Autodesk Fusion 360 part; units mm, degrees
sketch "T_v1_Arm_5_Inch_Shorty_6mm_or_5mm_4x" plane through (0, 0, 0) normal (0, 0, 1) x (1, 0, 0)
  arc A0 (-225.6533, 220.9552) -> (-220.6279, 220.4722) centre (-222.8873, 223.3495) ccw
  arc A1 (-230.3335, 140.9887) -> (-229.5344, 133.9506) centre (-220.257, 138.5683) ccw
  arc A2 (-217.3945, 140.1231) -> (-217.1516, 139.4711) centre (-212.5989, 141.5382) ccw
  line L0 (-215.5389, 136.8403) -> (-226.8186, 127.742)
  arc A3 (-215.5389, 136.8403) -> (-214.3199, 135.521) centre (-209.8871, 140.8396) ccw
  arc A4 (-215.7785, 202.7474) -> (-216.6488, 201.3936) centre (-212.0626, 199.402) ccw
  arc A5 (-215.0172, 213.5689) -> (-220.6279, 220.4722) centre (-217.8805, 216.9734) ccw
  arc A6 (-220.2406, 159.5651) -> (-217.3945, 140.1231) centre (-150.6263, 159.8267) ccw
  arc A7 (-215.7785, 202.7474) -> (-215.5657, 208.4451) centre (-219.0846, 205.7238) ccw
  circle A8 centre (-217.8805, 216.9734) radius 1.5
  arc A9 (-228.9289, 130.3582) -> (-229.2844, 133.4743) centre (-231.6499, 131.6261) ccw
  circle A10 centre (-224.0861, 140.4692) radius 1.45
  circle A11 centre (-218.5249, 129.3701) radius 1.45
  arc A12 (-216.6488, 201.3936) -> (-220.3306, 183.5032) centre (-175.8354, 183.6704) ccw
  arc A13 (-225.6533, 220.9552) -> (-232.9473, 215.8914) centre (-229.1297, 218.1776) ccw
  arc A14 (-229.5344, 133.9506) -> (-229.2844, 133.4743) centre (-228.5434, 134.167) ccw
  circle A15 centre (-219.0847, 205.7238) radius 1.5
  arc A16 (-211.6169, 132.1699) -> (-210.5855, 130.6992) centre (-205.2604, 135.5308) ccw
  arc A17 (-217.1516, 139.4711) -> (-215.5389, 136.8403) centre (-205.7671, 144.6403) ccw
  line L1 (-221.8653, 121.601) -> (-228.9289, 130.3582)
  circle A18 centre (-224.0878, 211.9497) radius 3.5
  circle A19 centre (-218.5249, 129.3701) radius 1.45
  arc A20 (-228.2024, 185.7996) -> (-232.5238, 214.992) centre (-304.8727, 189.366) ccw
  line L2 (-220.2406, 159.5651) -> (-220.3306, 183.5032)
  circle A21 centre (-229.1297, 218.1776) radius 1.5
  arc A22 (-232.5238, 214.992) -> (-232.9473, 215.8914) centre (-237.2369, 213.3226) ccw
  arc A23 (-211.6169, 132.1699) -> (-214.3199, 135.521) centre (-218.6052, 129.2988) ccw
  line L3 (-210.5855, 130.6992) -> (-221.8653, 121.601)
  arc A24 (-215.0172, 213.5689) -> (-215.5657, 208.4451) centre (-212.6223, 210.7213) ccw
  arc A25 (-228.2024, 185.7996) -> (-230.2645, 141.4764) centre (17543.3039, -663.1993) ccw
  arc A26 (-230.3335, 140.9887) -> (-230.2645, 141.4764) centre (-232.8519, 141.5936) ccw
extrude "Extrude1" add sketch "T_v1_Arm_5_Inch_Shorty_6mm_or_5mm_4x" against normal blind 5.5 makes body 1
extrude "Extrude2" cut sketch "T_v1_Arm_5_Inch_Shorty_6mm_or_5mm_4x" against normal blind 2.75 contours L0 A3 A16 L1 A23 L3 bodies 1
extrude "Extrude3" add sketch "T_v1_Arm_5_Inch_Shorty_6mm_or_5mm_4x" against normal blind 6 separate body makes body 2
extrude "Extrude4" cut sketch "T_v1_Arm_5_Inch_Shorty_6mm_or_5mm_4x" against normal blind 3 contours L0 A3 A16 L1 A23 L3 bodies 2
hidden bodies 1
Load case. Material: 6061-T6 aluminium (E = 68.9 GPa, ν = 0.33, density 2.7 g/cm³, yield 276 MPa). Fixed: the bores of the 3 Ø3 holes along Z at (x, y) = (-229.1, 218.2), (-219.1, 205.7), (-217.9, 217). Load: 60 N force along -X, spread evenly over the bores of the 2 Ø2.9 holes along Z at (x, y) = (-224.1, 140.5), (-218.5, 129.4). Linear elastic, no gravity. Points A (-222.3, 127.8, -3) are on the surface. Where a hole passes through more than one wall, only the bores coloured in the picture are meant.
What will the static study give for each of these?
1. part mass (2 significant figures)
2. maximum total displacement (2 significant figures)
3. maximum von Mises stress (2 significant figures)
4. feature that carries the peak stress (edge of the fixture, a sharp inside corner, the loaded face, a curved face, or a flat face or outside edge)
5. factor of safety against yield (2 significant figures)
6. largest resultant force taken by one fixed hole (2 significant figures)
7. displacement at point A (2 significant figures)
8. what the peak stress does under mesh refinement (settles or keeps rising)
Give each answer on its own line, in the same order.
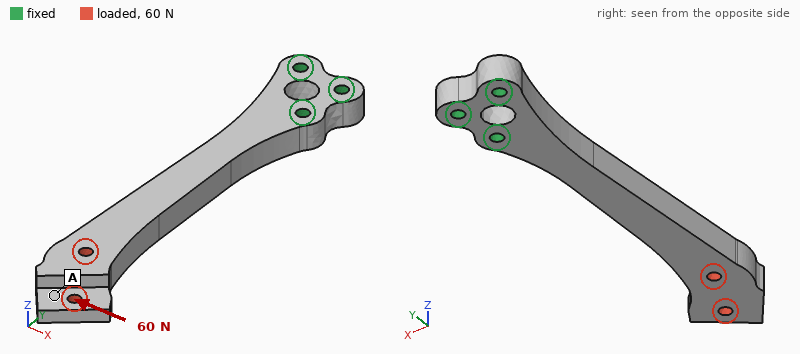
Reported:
16 g
0.35 mm
49 MPa
a curved face
5.7
300 N
0.31 mm
settles
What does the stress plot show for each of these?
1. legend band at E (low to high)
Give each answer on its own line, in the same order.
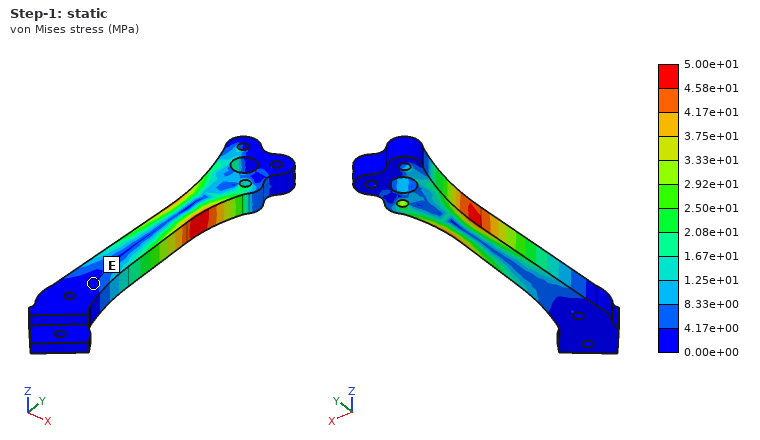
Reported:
0.00e+00 to 4.17e+00 MPa
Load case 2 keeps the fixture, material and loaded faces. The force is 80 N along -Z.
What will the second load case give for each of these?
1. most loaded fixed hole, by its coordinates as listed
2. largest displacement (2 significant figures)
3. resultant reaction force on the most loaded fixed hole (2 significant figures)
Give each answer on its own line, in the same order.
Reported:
(-219.1, 205.7)
1.0 mm
230 N
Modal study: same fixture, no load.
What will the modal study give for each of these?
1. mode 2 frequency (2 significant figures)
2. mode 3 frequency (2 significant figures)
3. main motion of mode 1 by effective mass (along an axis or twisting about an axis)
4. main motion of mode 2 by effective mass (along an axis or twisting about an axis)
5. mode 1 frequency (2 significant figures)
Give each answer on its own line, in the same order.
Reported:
1000 Hz
4400 Hz
along Z
along X
700 Hz
